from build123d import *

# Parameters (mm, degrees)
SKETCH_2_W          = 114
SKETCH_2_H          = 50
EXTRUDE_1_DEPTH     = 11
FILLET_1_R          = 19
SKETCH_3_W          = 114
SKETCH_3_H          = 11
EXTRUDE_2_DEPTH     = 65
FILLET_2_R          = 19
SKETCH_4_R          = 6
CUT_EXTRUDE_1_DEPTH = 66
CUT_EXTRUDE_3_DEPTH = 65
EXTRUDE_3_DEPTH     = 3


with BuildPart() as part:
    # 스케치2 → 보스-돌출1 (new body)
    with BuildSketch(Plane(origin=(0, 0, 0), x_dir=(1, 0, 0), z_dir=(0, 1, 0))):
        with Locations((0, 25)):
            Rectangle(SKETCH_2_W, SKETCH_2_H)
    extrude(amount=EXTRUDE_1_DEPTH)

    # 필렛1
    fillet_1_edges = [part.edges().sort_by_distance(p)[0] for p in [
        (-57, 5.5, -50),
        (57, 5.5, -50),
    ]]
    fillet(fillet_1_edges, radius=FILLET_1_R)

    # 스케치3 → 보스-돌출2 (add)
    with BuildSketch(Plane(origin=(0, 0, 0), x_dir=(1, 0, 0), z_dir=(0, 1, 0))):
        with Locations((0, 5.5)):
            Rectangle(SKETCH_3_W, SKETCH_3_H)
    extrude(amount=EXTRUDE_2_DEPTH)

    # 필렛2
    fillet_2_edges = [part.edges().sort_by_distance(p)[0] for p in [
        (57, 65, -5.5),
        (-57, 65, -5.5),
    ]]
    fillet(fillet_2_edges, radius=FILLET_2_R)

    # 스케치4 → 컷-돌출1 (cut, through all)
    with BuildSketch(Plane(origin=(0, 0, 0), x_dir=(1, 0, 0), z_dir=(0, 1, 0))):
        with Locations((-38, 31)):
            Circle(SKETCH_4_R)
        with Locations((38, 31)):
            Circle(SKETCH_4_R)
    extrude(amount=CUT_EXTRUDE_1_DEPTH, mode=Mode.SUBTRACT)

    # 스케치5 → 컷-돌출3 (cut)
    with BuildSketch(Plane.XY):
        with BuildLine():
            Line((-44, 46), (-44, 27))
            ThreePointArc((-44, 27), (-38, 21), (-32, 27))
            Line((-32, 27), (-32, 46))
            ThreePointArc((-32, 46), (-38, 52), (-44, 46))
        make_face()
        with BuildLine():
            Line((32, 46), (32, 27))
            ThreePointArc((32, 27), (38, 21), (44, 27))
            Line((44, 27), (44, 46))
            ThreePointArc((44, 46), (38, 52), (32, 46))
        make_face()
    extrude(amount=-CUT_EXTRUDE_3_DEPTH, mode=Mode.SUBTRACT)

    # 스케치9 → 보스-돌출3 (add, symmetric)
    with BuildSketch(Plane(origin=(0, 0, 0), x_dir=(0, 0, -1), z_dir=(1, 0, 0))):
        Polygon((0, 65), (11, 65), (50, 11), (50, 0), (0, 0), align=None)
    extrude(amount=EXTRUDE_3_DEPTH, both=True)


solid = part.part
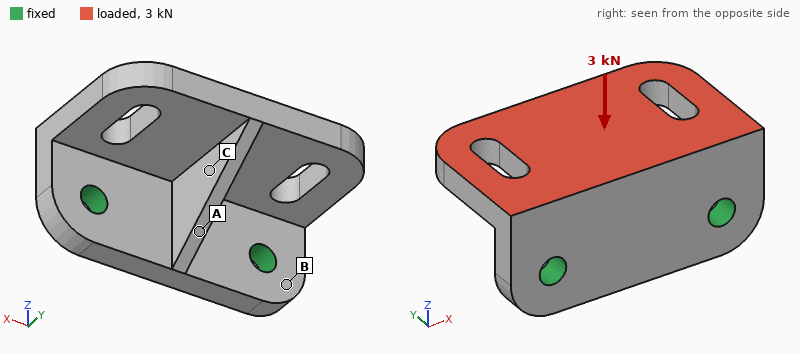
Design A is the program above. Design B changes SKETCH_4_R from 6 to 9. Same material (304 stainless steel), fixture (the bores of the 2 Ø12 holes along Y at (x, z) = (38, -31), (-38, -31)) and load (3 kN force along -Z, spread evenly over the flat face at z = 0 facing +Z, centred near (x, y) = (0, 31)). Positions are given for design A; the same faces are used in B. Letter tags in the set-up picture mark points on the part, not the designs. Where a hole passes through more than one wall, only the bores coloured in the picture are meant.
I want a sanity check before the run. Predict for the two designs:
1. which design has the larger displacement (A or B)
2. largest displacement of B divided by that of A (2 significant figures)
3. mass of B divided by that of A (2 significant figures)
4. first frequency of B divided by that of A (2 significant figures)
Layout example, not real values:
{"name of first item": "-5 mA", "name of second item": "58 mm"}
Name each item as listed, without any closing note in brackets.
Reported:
{"which design has the larger displacement": "A", "largest displacement of B divided by that of A": "0.80", "mass of B divided by that of A": "0.97", "first frequency of B divided by that of A": "1.2"}
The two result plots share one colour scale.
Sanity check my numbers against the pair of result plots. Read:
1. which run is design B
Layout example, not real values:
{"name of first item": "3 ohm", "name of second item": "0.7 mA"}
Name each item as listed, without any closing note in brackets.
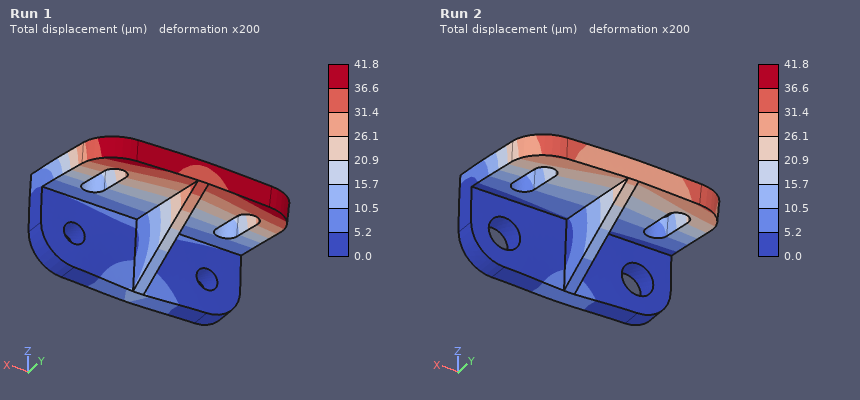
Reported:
{"which run is design B": "Run 2"}
